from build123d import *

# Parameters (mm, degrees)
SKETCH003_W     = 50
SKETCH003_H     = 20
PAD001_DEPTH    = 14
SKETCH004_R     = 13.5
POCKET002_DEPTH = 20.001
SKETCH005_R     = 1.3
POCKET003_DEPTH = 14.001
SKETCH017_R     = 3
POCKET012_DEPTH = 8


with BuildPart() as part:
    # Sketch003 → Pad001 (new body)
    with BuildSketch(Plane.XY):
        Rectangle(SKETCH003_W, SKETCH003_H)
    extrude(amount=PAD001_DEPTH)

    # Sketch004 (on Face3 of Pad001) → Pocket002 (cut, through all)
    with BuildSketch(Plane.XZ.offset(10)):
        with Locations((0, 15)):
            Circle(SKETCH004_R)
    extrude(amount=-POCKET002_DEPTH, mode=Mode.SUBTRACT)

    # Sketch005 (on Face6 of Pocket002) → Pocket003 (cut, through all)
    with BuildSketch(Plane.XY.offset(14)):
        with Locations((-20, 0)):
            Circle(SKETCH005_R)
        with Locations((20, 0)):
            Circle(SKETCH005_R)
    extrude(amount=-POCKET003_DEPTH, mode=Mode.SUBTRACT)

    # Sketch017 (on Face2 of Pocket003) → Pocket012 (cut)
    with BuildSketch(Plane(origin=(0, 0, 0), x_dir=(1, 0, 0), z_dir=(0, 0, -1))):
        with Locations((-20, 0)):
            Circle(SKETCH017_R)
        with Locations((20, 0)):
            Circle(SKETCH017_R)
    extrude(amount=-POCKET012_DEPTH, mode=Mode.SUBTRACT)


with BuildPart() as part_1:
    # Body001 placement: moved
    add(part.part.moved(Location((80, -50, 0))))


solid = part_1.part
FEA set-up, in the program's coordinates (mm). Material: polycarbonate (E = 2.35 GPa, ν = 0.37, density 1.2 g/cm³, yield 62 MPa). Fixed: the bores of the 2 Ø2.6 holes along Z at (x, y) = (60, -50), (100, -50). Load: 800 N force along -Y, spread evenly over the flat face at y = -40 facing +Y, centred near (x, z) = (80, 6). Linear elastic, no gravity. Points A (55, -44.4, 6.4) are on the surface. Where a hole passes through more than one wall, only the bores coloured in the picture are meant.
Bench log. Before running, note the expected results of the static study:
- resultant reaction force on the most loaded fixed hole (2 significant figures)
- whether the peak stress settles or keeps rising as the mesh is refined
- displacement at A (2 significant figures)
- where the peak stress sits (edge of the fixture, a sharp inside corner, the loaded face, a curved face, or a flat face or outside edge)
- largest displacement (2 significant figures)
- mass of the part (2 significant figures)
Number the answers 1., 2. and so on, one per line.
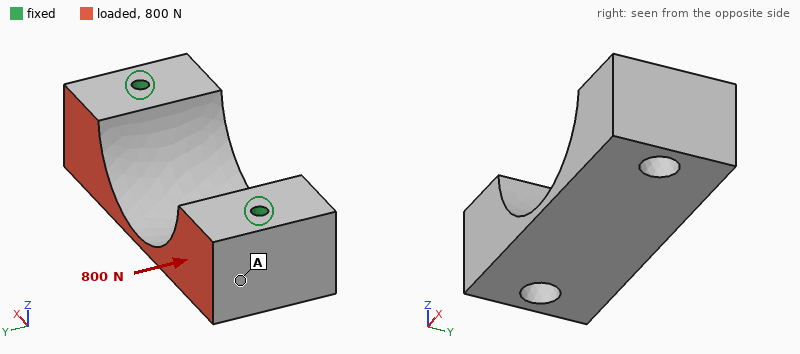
1. 400 N
2. keeps rising
3. 0.069 mm
4. edge of the fixture
5. 0.27 mm
6. 10.0 g
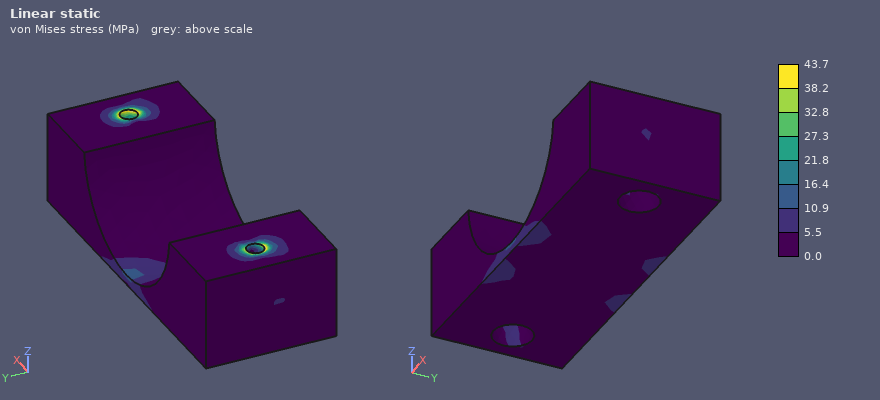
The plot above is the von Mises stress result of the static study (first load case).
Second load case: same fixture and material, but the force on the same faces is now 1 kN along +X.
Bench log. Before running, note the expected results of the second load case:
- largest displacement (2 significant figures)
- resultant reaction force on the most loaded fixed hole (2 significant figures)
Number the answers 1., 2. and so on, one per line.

1. 0.30 mm
2. 540 N
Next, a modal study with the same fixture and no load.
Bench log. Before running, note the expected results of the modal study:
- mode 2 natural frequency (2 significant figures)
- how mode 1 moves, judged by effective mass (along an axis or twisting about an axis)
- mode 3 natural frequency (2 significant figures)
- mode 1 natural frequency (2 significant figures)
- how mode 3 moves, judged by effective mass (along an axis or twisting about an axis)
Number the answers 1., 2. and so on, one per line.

1. 4200 Hz
2. along Y
3. 4400 Hz
4. 3300 Hz
5. along X
